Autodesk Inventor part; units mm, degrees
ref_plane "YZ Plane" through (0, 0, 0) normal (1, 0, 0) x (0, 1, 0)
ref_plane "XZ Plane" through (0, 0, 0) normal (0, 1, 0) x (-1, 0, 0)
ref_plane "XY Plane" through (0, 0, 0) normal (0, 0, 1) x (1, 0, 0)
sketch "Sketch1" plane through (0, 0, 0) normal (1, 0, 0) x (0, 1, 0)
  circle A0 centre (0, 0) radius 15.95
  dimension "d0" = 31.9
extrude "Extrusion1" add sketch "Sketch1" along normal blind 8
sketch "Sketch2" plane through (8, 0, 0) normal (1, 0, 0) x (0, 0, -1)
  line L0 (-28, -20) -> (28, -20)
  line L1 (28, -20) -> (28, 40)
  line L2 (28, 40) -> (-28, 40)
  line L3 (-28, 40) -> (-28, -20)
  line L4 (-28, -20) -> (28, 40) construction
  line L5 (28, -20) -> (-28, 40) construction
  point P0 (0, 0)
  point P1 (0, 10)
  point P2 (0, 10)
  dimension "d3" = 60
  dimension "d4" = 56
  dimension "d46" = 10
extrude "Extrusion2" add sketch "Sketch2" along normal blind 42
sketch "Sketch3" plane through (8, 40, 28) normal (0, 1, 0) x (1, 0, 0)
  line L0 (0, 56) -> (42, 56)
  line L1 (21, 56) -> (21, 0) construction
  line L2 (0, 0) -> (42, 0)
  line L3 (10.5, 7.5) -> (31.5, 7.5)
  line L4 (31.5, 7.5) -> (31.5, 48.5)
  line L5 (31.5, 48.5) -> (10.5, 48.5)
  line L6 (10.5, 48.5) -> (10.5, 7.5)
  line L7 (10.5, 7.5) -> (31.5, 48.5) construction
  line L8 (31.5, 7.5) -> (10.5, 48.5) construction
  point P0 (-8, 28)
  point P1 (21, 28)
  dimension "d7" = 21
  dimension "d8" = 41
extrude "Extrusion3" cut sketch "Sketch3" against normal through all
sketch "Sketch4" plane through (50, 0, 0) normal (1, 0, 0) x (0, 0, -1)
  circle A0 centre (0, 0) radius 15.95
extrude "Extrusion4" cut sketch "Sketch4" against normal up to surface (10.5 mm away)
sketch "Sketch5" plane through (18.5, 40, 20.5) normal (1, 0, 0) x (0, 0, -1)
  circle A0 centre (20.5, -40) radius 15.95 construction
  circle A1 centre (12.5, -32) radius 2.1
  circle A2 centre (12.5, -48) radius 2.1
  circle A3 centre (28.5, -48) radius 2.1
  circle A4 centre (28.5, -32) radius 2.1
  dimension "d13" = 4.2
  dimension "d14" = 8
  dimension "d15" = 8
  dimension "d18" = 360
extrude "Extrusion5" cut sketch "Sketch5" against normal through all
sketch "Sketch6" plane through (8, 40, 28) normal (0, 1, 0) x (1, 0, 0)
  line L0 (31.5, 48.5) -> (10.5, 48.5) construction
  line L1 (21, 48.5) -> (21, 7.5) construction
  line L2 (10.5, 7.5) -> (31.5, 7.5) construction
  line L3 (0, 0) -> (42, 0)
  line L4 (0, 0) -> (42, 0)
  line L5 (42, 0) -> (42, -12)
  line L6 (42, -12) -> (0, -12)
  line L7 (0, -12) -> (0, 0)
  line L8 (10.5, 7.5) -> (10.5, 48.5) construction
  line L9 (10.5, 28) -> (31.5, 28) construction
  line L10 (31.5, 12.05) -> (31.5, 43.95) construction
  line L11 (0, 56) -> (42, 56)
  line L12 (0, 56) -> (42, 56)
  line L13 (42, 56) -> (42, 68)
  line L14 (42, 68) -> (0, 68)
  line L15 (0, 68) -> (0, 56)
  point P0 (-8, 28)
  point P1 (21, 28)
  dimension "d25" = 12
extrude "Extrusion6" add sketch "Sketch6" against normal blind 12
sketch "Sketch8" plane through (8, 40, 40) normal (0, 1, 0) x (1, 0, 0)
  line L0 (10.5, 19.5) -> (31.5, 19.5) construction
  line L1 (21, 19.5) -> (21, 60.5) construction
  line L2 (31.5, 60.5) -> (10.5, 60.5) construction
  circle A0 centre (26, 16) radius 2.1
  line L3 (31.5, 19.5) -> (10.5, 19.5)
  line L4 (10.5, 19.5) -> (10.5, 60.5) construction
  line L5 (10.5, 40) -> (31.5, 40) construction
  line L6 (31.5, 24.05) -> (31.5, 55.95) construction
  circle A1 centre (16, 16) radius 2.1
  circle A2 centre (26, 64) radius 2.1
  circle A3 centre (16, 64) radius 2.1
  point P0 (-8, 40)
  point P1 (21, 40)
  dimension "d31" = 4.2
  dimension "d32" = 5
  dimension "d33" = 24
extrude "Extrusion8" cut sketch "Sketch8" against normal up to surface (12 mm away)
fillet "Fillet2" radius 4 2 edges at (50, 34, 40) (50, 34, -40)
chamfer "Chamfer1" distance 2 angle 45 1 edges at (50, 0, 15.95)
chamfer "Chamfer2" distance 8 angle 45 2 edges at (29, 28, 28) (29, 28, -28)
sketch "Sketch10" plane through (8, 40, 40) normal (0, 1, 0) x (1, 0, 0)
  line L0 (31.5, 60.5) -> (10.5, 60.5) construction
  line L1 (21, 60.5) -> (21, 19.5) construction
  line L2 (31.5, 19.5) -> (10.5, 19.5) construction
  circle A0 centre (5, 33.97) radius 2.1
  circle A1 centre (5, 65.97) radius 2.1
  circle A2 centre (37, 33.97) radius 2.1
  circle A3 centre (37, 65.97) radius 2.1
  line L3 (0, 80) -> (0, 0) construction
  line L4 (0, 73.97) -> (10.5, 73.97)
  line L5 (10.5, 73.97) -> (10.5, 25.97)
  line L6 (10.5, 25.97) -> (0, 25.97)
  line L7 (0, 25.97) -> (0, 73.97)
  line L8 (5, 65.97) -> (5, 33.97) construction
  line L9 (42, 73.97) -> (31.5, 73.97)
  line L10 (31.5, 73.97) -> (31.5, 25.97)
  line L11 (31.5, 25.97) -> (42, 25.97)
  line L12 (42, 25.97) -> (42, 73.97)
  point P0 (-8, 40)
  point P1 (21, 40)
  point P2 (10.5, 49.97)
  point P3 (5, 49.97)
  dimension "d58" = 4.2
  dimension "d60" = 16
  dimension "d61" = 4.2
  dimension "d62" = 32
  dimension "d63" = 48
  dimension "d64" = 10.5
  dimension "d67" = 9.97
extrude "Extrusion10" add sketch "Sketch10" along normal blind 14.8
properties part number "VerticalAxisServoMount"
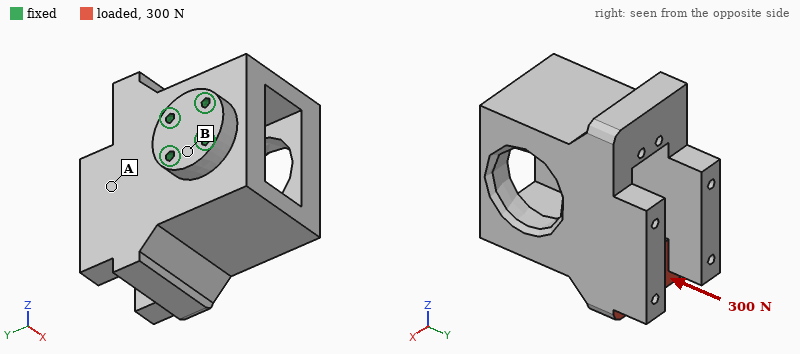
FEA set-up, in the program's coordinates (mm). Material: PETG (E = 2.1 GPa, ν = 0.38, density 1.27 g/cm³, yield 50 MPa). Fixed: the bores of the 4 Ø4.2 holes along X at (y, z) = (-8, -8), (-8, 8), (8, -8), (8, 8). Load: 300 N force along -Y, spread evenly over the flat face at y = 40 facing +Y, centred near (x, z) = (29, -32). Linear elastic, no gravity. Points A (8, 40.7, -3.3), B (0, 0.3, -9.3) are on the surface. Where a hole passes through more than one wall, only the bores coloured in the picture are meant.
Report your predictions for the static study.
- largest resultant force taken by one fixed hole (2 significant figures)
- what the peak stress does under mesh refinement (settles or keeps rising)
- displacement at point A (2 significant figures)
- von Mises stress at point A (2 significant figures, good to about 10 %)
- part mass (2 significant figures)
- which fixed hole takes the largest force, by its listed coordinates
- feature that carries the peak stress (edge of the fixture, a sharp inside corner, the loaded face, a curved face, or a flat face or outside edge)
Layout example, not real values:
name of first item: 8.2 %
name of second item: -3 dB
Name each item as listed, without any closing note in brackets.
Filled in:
largest resultant force taken by one fixed hole: 320 N
what the peak stress does under mesh refinement: keeps rising
displacement at point A: 0.066 mm
von Mises stress at point A: 0.70 MPa
part mass: 150 g
which fixed hole takes the largest force, by its listed coordinates: (8, -8)
feature that carries the peak stress: edge of the fixture
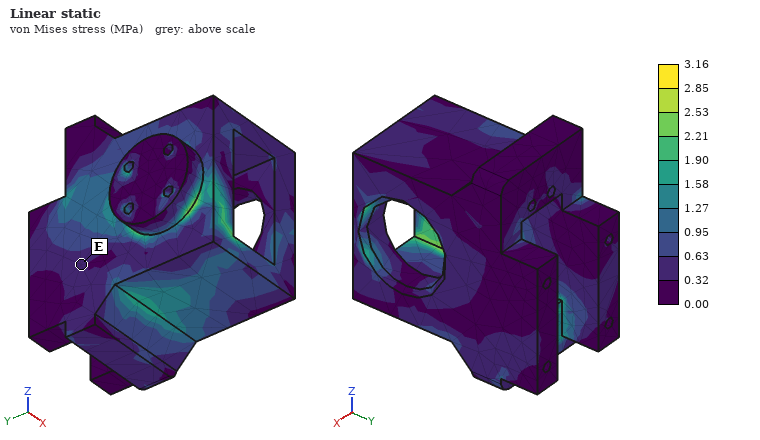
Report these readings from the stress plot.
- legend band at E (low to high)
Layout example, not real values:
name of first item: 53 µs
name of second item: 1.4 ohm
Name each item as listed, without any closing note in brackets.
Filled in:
legend band at E: 0.32 to 0.63 MPa
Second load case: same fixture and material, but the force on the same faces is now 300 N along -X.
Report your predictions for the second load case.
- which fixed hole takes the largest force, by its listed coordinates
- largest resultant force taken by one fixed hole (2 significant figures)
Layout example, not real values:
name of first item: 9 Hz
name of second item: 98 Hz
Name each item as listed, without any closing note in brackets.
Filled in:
which fixed hole takes the largest force, by its listed coordinates: (8, -8)
largest resultant force taken by one fixed hole: 440 N
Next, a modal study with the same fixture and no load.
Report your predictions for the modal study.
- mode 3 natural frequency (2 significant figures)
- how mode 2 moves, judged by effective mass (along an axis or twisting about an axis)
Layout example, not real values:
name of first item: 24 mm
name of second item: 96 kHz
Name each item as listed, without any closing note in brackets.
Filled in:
mode 3 natural frequency: 1200 Hz
how mode 2 moves, judged by effective mass: along Z
